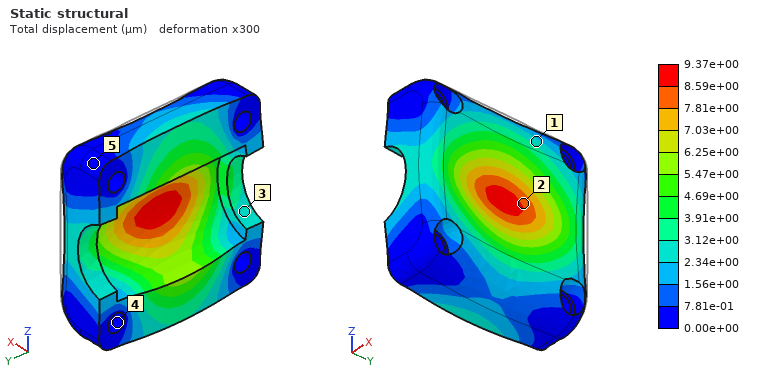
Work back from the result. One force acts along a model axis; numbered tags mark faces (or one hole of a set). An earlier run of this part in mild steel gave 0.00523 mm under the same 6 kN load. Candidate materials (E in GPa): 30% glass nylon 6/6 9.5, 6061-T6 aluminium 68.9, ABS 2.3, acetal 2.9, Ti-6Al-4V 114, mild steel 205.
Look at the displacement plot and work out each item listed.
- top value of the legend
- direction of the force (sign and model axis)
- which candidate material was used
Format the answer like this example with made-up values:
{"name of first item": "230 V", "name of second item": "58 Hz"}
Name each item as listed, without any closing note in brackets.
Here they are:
{"top value of the legend": "9.37e+00 µm", "direction of the force": "-X", "which candidate material was used": "Ti-6Al-4V"}
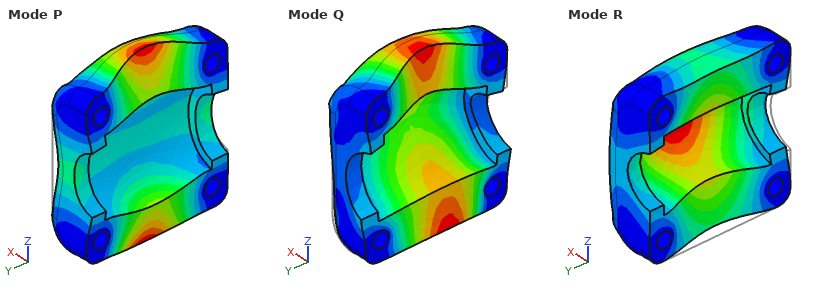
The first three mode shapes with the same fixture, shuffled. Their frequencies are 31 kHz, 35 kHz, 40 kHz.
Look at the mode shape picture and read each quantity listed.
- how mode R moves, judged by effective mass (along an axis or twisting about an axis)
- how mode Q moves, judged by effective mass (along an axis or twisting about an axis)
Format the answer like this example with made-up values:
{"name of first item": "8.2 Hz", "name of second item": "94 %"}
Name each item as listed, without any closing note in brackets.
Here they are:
{"how mode R moves, judged by effective mass": "along X", "how mode Q moves, judged by effective mass": "along Z"}
